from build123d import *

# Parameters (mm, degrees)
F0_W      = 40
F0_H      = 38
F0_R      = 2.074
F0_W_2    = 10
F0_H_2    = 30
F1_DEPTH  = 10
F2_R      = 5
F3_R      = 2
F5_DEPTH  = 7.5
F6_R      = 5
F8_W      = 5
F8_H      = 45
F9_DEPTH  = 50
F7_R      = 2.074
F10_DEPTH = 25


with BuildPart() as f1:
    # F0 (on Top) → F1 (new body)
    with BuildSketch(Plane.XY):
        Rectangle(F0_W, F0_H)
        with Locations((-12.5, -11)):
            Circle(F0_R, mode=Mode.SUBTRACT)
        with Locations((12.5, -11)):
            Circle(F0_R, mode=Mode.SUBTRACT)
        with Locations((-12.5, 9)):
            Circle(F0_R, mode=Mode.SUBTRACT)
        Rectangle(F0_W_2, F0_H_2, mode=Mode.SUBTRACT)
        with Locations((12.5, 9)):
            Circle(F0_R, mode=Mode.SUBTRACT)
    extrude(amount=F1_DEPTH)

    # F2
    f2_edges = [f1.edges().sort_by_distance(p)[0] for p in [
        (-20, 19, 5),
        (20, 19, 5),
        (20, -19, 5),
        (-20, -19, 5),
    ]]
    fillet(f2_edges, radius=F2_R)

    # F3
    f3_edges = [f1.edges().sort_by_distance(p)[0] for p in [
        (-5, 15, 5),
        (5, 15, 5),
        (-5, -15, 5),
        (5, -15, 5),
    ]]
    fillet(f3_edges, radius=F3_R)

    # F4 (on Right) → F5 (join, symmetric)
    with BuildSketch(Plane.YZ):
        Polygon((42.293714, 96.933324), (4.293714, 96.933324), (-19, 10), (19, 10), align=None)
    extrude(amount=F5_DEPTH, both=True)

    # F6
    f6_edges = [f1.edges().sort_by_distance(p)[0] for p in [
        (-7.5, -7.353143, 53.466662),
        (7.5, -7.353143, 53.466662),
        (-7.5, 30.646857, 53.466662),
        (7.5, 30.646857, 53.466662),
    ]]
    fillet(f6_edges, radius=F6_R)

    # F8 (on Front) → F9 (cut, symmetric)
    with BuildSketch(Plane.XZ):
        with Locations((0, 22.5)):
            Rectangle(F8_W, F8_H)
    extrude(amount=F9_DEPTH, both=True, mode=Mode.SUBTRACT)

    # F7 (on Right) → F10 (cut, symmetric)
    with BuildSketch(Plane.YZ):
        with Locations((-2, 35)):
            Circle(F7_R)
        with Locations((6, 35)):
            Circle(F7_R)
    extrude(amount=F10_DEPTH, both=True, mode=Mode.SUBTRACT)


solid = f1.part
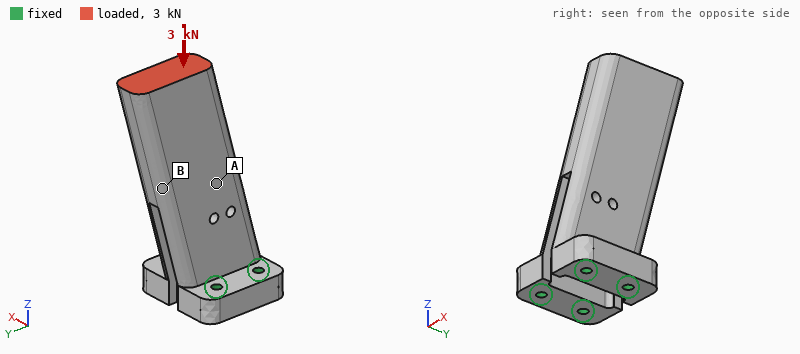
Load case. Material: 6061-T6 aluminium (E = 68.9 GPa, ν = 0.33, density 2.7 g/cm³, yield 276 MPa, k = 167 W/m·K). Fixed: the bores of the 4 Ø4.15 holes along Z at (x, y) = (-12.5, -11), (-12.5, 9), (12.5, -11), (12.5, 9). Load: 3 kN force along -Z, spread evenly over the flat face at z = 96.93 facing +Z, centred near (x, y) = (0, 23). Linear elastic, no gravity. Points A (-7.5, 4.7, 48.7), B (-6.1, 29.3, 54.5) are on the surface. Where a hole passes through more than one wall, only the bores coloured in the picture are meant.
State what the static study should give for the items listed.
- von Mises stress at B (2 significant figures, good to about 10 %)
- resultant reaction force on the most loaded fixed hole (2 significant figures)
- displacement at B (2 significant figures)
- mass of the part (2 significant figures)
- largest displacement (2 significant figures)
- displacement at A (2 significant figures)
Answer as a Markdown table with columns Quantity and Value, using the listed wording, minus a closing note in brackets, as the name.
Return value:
| Quantity | Value |
|---|---|
| von Mises stress at B | 15 MPa |
| resultant reaction force on the most loaded fixed hole | 2.1 kN |
| displacement at B | 0.072 mm |
| mass of the part | 140 g |
| largest displacement | 0.15 mm |
| displacement at A | 0.044 mm |
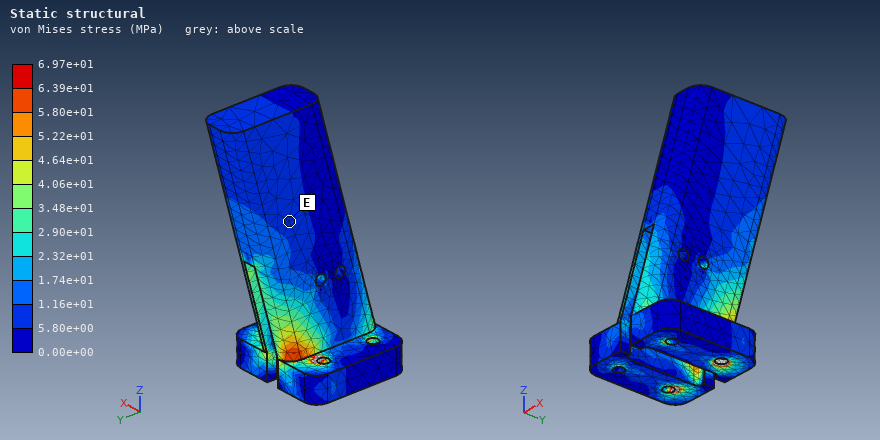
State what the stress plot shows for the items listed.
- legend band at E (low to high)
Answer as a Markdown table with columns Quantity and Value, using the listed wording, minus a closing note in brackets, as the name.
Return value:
| Quantity | Value |
|---|---|
| legend band at E | 5.80e+00 to 1.16e+01 MPa |
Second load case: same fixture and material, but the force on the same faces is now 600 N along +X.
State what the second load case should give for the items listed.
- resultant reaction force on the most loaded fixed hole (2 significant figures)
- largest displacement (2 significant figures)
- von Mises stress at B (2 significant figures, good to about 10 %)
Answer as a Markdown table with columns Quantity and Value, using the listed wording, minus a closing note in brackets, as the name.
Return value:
| Quantity | Value |
|---|---|
| resultant reaction force on the most loaded fixed hole | 2.1 kN |
| largest displacement | 0.40 mm |
| von Mises stress at B | 18 MPa |
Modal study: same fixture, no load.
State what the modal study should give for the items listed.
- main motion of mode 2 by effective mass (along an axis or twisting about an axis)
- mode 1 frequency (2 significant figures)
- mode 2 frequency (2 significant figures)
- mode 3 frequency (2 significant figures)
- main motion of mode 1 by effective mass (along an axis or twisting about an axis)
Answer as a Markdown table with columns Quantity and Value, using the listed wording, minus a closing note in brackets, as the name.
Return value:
| Quantity | Value |
|---|---|
| main motion of mode 2 by effective mass | along Y |
| mode 1 frequency | 1000 Hz |
| mode 2 frequency | 1900 Hz |
| mode 3 frequency | 3100 Hz |
| main motion of mode 1 by effective mass | along X |
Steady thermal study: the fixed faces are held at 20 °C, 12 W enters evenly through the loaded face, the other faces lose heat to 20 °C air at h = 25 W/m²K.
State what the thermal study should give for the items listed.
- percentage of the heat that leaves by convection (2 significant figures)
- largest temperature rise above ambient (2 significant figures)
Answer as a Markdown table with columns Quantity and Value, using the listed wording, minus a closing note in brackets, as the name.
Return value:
| Quantity | Value |
|---|---|
| percentage of the heat that leaves by convection | 18 % |
| largest temperature rise above ambient | 15 K |
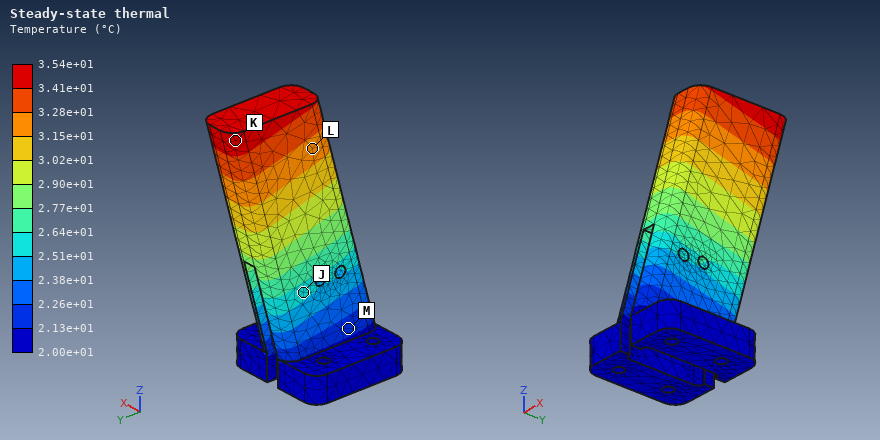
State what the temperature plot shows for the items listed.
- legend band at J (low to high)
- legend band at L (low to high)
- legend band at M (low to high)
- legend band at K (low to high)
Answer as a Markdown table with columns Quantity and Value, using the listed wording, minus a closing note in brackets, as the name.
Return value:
| Quantity | Value |
|---|---|
| legend band at J | 2.51e+01 to 2.64e+01 °C |
| legend band at L | 3.15e+01 to 3.28e+01 °C |
| legend band at M | 2.13e+01 to 2.26e+01 °C |
| legend band at K | 3.41e+01 to 3.54e+01 °C |
